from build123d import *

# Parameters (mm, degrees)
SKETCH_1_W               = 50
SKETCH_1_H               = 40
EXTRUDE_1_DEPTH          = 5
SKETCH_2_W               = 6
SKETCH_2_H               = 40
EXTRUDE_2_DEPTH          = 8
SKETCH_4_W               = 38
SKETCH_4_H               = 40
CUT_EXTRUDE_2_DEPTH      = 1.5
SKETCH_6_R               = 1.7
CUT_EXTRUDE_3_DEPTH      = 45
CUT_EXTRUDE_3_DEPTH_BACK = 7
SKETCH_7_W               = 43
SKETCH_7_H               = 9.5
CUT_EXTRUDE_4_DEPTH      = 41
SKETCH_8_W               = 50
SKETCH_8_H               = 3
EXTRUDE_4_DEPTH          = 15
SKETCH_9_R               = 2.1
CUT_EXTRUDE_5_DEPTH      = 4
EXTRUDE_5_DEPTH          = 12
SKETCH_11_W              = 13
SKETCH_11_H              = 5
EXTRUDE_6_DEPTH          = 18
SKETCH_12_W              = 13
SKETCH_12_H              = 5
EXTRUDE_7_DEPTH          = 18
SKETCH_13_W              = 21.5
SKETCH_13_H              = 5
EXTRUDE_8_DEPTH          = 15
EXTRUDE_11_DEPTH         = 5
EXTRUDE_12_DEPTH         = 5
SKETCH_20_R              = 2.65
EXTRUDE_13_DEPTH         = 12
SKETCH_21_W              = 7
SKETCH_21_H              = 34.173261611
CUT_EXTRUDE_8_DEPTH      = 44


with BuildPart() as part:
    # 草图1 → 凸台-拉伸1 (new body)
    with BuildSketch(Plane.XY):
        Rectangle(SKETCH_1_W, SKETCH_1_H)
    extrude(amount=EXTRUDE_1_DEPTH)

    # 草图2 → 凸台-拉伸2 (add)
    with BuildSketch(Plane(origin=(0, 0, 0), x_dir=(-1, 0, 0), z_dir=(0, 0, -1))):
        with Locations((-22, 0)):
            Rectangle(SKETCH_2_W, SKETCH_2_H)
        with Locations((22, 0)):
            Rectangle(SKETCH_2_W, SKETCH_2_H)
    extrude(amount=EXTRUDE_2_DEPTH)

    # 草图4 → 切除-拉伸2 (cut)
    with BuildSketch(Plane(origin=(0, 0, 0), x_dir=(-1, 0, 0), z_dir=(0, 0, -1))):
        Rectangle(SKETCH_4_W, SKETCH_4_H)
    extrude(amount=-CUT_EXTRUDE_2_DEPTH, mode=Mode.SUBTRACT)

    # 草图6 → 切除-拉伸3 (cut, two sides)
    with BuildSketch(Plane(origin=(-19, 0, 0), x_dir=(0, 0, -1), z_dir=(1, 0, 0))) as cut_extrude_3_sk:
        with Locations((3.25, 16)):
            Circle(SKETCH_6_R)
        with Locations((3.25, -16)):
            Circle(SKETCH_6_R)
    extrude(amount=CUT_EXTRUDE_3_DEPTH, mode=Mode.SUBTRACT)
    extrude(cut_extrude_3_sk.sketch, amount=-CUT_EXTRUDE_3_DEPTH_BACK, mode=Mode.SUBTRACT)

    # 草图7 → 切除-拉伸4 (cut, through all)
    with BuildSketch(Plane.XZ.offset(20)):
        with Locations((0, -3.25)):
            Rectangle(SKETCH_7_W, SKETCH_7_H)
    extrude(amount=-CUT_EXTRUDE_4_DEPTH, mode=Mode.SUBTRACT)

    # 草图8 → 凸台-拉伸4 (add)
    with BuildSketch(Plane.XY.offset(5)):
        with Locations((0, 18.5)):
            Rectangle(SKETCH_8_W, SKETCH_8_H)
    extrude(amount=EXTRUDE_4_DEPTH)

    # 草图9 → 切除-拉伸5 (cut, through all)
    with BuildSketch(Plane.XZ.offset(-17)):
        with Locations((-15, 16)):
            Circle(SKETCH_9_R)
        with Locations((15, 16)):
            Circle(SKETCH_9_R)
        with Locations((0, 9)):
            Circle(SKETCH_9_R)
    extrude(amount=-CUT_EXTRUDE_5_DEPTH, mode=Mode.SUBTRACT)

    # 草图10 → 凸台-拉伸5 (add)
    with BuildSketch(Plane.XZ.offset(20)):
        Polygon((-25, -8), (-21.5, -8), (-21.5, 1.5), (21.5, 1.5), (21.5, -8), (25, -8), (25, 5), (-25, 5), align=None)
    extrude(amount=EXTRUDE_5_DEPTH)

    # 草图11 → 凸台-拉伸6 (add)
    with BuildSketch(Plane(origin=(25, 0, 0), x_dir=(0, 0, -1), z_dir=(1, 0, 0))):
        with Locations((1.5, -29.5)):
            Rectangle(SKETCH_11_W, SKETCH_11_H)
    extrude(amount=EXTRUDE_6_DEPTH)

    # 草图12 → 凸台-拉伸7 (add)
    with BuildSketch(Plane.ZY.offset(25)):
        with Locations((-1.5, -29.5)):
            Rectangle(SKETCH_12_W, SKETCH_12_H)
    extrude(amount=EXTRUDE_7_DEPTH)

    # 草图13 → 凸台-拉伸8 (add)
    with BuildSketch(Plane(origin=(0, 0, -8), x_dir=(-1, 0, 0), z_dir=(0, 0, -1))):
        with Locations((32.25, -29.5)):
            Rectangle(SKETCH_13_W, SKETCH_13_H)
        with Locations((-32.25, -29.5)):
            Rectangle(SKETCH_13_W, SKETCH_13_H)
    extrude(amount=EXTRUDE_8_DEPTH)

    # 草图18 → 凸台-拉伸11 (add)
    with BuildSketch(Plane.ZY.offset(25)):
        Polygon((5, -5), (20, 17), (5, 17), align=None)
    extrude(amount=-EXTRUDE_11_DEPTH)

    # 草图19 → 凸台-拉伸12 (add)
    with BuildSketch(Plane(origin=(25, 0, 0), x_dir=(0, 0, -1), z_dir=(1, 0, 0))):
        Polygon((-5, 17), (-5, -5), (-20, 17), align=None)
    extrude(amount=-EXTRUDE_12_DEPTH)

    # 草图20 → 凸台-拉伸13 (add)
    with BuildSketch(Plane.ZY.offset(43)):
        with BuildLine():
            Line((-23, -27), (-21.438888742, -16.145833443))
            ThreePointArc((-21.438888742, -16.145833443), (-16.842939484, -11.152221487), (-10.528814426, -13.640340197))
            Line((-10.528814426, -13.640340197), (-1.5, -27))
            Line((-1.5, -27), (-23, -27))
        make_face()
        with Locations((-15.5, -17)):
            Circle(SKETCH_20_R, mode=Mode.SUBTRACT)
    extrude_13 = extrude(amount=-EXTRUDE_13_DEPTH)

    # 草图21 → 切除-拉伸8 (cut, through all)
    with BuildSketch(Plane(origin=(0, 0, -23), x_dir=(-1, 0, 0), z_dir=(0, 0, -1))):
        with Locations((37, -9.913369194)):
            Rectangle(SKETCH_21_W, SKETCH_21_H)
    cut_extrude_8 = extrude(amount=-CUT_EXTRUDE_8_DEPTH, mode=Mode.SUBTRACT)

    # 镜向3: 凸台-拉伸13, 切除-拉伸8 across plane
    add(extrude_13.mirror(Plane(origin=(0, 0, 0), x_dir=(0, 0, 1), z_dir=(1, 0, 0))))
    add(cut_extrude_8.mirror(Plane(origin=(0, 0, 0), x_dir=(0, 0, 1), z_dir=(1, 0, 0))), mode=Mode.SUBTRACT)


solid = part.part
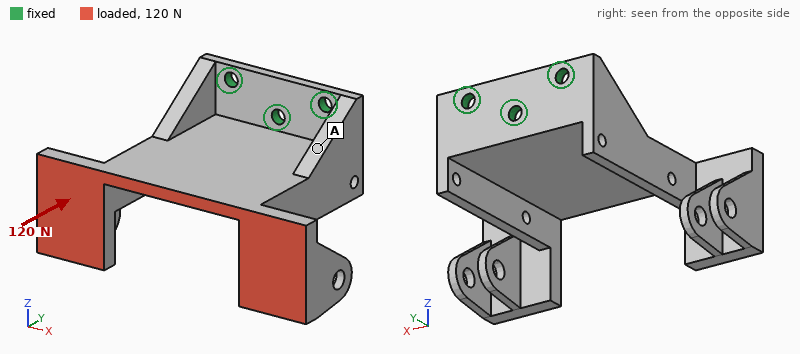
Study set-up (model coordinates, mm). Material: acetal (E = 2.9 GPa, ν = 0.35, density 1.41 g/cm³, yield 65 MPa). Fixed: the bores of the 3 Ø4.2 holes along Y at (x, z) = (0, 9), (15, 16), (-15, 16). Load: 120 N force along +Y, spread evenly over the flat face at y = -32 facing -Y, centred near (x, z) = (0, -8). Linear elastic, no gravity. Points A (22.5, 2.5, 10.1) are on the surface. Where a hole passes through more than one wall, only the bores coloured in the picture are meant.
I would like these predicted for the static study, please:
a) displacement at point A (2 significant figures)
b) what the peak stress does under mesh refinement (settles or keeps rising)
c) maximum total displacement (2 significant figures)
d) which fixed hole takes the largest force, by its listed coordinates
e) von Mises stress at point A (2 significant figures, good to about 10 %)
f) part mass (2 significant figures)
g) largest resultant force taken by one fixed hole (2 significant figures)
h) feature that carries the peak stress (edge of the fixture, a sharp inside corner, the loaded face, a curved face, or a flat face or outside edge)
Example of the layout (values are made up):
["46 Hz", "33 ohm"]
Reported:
["0.18 mm", "keeps rising", "1.1 mm", "(0, 9)", "2.9 MPa", "34 g", "200 N", "edge of the fixture"]
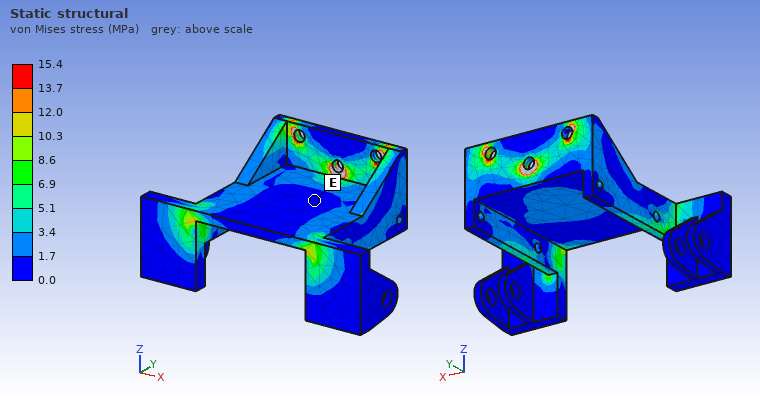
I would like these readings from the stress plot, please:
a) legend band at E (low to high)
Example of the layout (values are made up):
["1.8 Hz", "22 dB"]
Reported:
["0.0 to 1.7 MPa"]
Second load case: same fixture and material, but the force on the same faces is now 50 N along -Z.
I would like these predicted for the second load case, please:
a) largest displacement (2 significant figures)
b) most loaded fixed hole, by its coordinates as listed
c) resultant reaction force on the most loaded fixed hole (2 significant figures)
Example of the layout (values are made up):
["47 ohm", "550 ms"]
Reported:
["1.3 mm", "(0, 9)", "180 N"]
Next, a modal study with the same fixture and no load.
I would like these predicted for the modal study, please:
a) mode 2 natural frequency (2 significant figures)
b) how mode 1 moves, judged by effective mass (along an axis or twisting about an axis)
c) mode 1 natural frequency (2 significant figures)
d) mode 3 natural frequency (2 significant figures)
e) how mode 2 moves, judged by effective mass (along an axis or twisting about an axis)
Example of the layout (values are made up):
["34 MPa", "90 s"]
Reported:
["290 Hz", "twisting about Y", "250 Hz", "430 Hz", "along Z"]
